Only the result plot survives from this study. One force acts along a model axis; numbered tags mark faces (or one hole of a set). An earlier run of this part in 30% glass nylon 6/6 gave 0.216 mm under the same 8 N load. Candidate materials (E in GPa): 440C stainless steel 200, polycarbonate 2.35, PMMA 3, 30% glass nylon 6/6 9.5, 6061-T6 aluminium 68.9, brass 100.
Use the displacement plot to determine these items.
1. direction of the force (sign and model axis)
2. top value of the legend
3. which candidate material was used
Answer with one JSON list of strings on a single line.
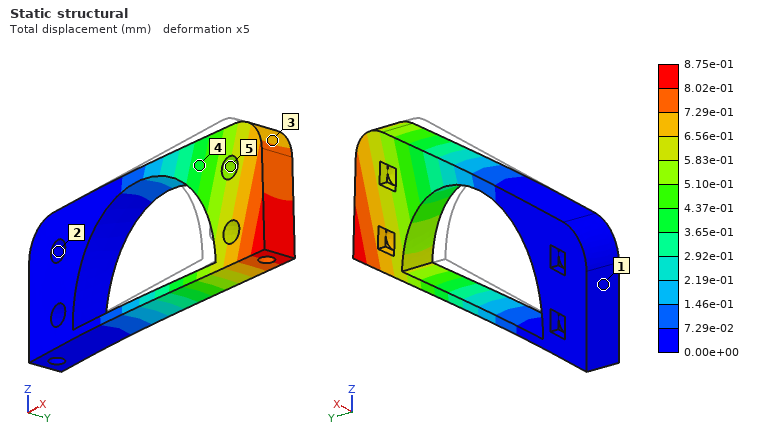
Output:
["+Y", "8.75e-01 mm", "polycarbonate"]
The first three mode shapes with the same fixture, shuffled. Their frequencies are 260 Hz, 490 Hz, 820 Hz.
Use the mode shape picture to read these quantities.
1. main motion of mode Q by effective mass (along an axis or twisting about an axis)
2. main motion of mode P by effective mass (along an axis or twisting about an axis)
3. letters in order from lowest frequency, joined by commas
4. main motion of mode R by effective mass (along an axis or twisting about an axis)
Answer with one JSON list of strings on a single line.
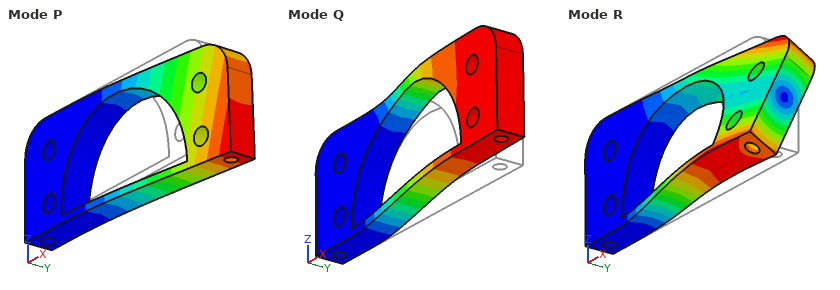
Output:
["along Z", "along Y", "P, Q, R", "twisting about X"]
